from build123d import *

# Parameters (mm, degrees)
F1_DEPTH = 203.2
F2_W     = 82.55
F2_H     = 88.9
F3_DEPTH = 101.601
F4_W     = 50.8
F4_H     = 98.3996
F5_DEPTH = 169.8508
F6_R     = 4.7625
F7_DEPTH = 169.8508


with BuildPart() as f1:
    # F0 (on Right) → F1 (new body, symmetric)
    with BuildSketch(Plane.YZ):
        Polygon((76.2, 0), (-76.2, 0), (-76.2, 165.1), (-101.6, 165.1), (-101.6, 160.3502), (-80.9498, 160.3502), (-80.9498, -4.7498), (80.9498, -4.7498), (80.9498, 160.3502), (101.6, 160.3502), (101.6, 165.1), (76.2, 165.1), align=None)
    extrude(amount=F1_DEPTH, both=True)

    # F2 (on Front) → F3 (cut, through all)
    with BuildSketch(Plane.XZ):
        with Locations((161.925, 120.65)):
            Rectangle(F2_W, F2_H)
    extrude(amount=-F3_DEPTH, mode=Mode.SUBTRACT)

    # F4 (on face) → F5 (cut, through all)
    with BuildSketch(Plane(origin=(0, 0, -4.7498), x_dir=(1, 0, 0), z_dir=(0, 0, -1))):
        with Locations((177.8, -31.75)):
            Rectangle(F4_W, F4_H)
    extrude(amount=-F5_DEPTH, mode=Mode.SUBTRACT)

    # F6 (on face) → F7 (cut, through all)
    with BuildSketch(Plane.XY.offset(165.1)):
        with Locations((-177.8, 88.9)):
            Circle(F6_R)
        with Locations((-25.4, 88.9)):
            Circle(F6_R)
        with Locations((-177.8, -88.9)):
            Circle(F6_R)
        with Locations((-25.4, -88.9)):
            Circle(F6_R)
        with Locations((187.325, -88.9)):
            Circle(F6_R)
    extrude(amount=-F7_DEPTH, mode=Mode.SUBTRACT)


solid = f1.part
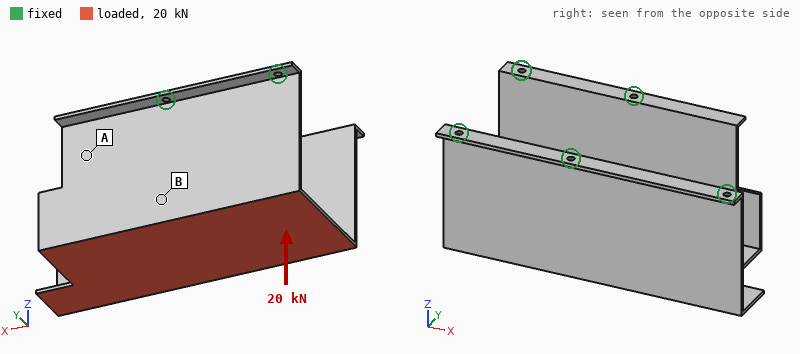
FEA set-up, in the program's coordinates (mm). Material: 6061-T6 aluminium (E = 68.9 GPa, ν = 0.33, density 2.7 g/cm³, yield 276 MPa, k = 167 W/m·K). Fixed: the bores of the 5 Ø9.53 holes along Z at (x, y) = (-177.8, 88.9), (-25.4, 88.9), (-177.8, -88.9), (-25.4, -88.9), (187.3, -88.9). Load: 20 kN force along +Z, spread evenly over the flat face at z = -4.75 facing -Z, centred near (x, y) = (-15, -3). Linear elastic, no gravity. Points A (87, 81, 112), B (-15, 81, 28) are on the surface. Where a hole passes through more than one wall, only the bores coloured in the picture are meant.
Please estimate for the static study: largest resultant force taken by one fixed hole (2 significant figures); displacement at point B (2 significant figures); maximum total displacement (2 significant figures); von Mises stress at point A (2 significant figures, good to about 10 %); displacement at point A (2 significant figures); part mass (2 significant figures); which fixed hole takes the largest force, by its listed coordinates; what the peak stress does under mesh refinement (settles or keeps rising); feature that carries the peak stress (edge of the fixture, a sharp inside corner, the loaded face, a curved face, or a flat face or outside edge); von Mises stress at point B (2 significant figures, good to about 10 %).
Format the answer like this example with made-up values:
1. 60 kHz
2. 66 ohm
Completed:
1. 9.1 kN
2. 0.98 mm
3. 2.6 mm
4. 26 MPa
5. 0.93 mm
6. 2.5 kg
7. (-25.4, 88.9)
8. keeps rising
9. edge of the fixture
10. 76 MPa
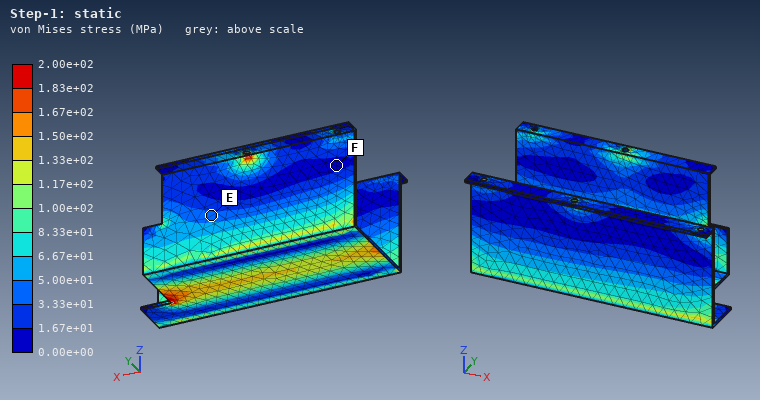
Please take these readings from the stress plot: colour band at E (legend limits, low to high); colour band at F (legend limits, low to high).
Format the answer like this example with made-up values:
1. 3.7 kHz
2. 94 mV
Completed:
1. 3.33e+01 to 5.00e+01 MPa
2. 0.00e+00 to 1.67e+01 MPa
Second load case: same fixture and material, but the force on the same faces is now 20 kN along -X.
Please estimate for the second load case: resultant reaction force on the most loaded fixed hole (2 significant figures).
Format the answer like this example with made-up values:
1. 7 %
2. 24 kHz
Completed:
1. 11 kN
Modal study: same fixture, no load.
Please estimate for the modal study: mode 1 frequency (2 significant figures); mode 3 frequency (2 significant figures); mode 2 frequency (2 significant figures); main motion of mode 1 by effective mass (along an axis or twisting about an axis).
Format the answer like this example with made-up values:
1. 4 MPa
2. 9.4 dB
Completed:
1. 110 Hz
2. 510 Hz
3. 460 Hz
4. along Y
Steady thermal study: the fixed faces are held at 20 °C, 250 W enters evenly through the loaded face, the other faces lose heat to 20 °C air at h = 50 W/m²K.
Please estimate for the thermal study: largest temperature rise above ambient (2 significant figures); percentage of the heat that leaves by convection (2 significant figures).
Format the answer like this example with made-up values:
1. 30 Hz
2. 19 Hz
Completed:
1. 33 K
2. 90 %
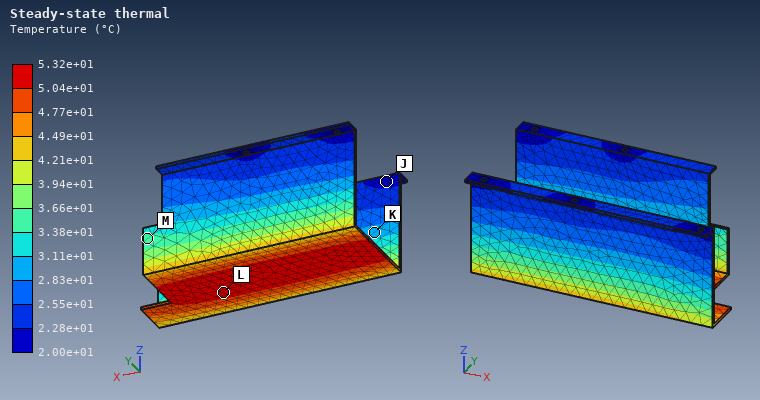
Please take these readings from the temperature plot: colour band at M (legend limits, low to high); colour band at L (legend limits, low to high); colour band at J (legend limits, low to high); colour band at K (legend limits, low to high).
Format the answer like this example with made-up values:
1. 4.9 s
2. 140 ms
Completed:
1. 3.38e+01 to 3.66e+01 °C
2. 5.04e+01 to 5.32e+01 °C
3. 2.00e+01 to 2.28e+01 °C
4. 2.83e+01 to 3.11e+01 °C
